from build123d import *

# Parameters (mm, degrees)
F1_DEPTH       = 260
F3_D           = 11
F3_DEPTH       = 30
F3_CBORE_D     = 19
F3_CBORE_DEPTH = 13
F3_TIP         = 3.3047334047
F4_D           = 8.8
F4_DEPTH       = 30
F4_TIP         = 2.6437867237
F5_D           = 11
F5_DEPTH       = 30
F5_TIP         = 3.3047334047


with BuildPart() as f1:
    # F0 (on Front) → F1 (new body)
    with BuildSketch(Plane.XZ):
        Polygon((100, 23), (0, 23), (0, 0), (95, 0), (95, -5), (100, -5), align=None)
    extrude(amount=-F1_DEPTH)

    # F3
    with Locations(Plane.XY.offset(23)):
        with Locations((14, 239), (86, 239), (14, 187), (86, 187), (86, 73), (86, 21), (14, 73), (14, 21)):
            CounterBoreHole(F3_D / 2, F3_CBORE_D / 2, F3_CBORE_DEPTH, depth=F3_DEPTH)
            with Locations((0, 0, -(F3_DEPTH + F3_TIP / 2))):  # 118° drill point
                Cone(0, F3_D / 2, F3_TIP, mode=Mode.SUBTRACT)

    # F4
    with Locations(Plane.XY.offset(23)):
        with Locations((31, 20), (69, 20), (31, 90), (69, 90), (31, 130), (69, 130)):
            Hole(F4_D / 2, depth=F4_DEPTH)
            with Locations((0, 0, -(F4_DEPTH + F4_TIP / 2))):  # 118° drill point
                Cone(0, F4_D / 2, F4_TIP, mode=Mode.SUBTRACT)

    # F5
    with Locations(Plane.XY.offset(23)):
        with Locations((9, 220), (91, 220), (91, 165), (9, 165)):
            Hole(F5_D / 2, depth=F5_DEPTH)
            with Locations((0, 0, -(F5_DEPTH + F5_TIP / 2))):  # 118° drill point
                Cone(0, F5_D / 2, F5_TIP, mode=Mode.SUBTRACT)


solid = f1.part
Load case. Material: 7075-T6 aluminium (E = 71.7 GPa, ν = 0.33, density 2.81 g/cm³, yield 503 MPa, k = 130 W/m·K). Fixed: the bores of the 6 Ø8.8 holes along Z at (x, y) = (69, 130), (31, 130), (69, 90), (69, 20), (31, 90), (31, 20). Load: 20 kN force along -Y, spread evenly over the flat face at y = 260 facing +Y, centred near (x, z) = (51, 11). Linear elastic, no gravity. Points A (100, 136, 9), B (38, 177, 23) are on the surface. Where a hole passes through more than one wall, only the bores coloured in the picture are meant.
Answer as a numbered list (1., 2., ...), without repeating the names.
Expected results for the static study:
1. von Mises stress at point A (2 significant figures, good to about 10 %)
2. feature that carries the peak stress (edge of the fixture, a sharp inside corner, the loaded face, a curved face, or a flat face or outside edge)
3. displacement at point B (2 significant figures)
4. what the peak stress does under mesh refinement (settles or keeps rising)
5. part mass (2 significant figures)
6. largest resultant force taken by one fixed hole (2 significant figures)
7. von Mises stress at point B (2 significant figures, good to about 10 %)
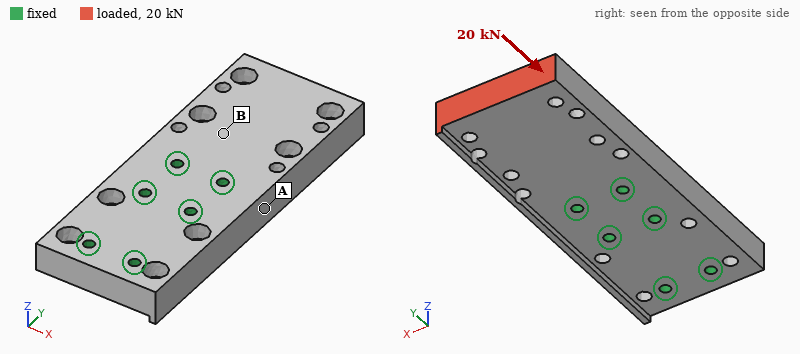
1. 4.8 MPa
2. a sharp inside corner
3. 7.7 µm
4. keeps rising
5. 1.5 kg
6. 8.2 kN
7. 13 MPa
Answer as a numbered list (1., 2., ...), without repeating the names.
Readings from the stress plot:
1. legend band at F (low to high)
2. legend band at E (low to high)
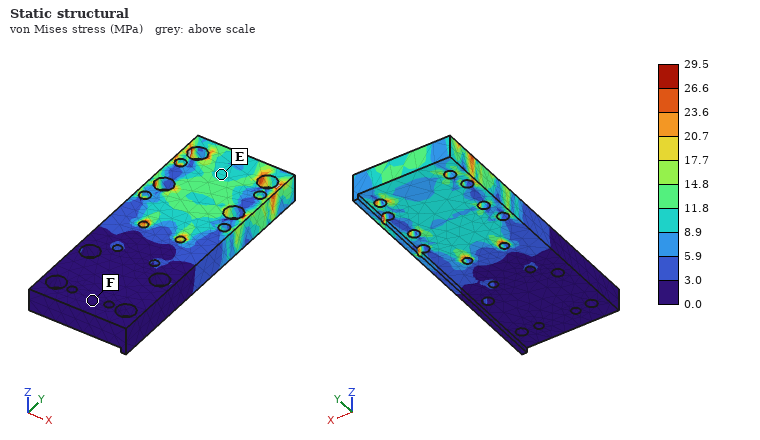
1. 0.0 to 3.0 MPa
2. 8.9 to 11.8 MPa
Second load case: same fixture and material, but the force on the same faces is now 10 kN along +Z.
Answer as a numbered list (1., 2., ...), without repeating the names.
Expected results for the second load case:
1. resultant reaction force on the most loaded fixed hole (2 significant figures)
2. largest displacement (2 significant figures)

1. 11 kN
2. 1.2 mm
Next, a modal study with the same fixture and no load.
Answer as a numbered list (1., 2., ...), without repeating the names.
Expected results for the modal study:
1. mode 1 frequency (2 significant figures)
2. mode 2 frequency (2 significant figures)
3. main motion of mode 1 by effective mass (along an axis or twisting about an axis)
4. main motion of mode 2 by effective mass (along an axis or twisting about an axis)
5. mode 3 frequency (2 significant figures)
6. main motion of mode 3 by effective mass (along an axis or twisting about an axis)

1. 1100 Hz
2. 2800 Hz
3. along Z
4. twisting about Y
5. 2900 Hz
6. along X
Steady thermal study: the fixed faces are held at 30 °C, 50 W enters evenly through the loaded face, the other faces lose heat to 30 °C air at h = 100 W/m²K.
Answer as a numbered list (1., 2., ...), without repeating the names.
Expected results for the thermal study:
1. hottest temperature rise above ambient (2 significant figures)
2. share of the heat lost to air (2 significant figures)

1. 17 K
2. 56 %
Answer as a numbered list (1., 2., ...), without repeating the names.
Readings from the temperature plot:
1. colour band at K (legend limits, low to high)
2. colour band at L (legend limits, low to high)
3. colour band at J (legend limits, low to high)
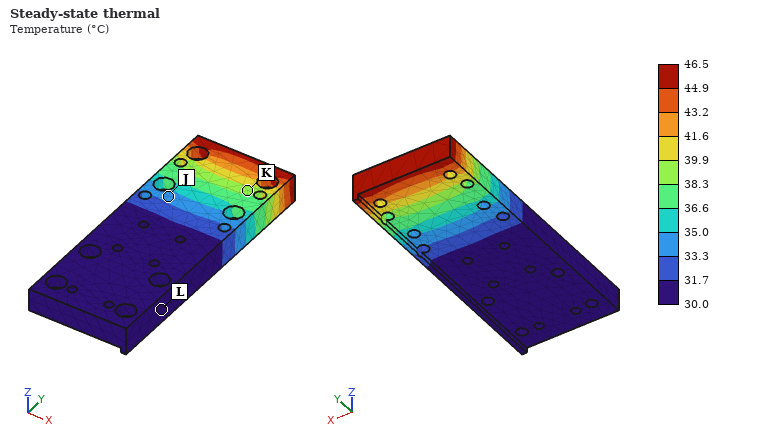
1. 38.3 to 39.9 °C
2. 30.0 to 31.7 °C
3. 33.3 to 35.0 °C
